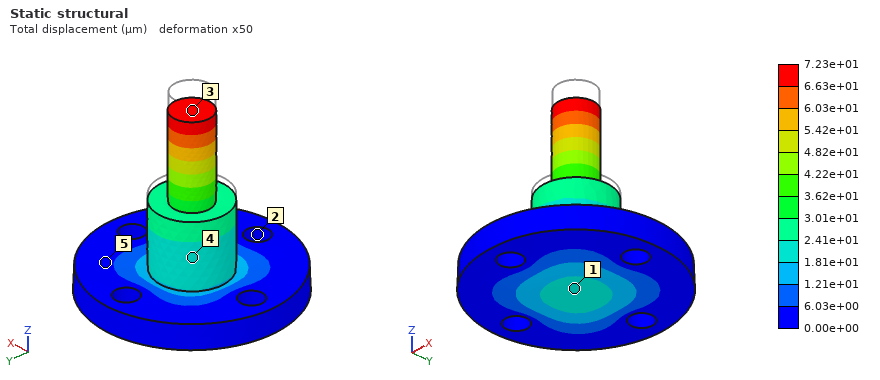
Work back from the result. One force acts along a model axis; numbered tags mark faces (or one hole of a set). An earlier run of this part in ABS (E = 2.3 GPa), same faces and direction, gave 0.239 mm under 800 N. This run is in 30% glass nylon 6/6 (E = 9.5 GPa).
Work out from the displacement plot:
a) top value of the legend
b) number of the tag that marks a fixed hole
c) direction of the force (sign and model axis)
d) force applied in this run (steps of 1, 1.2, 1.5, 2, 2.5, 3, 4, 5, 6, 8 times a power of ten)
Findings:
7.23e+01 µm
2
-Z
1 kN
